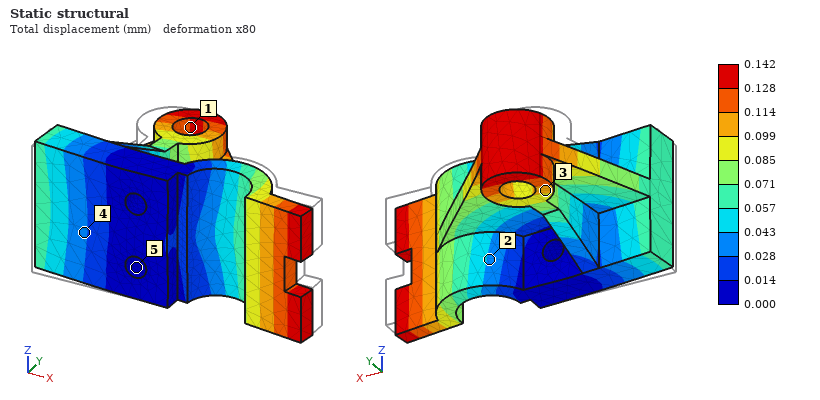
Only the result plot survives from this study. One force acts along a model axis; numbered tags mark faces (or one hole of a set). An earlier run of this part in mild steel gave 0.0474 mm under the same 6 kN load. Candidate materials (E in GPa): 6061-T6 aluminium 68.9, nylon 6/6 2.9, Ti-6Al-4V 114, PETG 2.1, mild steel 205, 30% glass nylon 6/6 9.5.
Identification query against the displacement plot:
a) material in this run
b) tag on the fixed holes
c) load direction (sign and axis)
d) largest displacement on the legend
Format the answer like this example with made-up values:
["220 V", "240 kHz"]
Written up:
["6061-T6 aluminium", "5", "+X", "0.142 mm"]
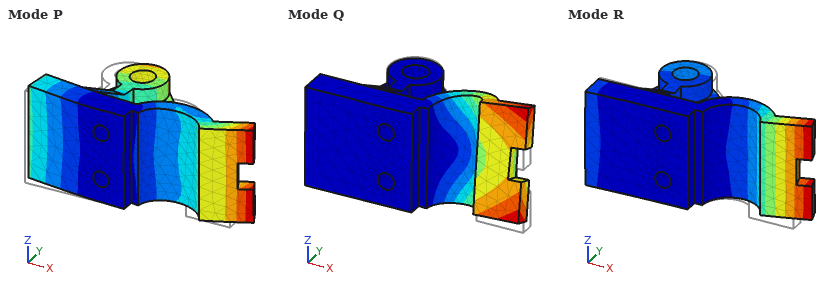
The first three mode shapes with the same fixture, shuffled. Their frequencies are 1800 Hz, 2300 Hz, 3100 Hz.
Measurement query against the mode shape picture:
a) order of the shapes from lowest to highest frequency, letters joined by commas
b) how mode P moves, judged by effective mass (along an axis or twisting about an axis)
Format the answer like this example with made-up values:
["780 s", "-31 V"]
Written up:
["R, Q, P", "along X"]
